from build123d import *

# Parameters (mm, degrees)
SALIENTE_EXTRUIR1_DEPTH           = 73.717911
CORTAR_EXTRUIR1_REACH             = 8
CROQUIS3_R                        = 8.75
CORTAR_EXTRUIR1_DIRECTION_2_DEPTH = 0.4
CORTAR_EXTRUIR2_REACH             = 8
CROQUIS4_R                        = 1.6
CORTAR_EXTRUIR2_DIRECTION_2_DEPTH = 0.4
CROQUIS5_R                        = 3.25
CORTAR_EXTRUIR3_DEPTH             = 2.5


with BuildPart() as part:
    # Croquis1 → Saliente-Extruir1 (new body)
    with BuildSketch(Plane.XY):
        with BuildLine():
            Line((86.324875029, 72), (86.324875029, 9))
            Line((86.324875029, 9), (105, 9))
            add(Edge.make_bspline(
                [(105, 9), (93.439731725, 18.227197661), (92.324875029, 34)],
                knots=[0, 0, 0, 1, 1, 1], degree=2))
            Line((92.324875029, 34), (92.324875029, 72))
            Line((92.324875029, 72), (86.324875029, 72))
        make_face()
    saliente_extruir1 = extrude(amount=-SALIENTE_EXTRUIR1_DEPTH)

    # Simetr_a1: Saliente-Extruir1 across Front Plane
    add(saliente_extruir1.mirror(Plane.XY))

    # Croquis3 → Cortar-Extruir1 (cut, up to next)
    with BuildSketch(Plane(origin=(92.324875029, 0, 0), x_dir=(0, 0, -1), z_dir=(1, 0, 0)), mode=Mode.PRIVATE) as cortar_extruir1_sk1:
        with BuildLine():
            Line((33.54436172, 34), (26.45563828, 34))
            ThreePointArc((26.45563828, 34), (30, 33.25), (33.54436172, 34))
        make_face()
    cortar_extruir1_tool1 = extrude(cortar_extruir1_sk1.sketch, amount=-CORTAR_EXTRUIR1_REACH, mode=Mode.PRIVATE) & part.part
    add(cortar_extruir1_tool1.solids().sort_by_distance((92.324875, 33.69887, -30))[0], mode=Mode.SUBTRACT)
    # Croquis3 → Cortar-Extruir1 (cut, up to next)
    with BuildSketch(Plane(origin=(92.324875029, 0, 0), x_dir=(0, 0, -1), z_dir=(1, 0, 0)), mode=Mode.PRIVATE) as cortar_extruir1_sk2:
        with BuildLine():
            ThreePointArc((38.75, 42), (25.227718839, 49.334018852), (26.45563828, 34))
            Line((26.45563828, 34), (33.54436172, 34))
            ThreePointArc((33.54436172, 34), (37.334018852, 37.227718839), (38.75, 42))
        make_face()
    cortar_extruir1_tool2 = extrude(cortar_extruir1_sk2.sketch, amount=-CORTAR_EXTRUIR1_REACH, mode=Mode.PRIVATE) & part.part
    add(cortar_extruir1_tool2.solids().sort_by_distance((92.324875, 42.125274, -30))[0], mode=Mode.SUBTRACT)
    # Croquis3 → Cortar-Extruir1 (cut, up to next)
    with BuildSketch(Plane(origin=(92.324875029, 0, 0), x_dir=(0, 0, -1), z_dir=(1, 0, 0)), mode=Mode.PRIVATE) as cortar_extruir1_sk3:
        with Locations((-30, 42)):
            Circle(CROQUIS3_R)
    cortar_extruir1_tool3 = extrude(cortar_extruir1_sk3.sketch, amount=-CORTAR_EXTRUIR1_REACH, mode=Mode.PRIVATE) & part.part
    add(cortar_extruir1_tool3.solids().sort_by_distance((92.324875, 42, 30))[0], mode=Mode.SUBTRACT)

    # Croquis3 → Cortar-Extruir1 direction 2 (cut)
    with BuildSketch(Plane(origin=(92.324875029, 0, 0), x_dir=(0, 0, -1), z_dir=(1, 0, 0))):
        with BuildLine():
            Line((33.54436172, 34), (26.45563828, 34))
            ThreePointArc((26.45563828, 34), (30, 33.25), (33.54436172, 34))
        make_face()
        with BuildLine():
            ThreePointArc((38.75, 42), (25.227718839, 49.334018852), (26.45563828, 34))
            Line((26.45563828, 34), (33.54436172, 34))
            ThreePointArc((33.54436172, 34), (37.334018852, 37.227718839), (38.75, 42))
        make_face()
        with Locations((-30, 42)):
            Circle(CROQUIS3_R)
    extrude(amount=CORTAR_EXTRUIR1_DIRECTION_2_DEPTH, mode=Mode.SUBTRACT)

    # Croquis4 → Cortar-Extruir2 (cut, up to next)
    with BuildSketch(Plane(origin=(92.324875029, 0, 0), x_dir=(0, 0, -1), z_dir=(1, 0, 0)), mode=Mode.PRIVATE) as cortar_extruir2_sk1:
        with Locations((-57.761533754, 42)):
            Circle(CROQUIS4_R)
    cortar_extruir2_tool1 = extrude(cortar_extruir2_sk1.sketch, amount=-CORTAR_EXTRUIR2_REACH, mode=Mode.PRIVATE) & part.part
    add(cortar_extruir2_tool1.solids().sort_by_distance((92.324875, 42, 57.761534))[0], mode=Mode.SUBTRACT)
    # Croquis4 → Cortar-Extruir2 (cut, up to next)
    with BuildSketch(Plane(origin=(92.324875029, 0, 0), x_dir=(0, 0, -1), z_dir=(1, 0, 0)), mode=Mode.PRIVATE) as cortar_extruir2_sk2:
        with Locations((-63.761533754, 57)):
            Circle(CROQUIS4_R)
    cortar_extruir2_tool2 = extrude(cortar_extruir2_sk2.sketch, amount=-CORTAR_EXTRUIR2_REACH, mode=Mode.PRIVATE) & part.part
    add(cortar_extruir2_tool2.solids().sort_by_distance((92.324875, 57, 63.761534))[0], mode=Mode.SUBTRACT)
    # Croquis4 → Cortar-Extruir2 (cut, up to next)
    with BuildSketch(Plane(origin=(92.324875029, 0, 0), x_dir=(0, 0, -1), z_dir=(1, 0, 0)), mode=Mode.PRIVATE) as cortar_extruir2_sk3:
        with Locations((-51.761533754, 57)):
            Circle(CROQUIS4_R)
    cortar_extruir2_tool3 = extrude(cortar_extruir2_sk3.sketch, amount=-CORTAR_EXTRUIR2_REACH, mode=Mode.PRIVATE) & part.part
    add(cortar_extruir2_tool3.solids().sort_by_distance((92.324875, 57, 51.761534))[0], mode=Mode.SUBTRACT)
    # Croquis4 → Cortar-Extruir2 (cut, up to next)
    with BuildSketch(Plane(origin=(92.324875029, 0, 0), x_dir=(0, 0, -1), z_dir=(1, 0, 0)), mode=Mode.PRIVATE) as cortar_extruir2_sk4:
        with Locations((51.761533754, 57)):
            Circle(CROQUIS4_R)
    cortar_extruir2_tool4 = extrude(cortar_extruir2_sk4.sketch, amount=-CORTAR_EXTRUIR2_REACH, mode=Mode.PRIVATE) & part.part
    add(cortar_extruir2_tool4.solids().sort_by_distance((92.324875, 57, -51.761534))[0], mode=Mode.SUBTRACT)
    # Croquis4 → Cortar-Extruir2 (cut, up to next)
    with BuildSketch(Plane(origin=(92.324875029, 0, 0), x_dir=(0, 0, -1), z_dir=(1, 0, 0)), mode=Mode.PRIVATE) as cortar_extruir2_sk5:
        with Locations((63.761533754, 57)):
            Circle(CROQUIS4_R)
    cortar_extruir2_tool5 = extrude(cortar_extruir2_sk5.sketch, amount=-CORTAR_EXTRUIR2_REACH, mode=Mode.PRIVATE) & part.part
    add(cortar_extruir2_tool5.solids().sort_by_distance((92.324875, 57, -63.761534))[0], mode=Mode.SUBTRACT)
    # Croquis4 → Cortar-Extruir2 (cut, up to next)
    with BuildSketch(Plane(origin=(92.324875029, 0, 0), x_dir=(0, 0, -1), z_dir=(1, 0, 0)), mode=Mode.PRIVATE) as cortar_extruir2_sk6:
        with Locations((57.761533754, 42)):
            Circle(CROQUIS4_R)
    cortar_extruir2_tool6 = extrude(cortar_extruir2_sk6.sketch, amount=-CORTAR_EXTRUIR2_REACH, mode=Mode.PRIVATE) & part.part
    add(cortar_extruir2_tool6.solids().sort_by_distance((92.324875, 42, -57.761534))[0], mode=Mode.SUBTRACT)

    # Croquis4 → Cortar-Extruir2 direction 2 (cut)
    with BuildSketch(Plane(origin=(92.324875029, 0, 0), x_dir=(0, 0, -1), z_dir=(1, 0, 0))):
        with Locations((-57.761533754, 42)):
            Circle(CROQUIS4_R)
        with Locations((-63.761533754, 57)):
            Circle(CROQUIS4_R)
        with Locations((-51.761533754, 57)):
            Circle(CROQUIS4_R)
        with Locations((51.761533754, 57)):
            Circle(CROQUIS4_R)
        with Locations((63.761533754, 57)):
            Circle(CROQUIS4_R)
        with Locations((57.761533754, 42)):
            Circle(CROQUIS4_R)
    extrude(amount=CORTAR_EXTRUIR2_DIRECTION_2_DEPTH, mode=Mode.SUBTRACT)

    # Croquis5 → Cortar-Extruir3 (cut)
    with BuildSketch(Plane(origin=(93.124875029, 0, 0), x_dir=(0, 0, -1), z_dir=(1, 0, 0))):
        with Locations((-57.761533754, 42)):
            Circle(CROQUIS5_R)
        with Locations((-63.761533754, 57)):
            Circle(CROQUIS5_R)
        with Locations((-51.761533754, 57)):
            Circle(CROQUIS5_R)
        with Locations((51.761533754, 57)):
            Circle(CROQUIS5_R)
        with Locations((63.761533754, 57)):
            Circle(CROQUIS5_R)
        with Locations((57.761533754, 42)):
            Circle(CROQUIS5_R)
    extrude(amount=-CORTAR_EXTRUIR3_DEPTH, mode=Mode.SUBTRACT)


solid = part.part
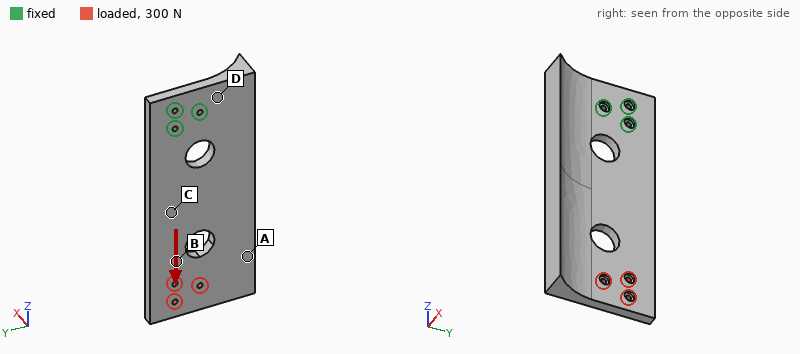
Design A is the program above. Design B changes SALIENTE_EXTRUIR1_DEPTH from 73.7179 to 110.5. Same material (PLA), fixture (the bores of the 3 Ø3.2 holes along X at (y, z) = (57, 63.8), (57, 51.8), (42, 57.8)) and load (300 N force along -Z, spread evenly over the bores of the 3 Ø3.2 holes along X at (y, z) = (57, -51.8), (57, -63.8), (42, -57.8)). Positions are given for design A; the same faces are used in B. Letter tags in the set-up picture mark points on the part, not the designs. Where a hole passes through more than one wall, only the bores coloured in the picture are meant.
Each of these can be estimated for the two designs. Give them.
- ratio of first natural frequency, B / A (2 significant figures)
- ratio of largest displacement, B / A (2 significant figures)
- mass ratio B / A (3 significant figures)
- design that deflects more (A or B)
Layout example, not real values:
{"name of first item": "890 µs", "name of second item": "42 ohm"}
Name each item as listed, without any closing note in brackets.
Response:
{"ratio of first natural frequency, B / A": "0.70", "ratio of largest displacement, B / A": "1.3", "mass ratio B / A": "1.52", "design that deflects more": "B"}
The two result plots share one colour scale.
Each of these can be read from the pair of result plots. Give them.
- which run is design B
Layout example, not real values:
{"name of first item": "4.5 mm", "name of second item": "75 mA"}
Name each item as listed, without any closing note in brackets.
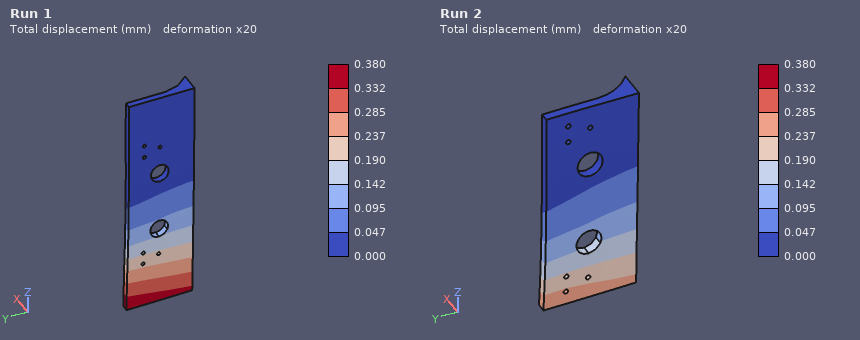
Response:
{"which run is design B": "Run 1"}
